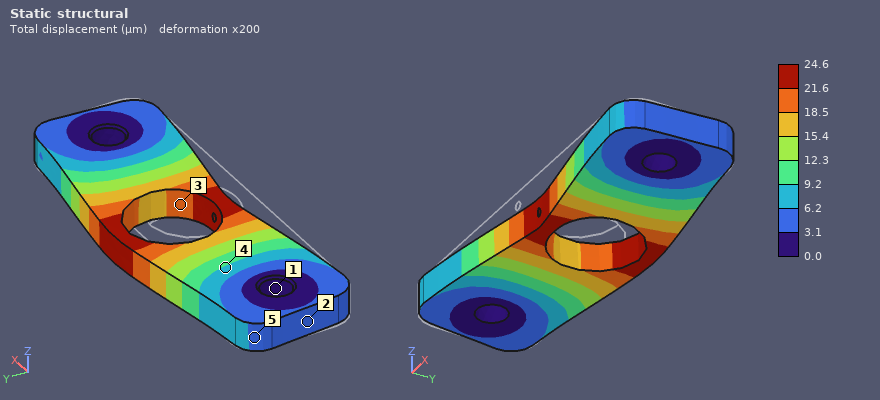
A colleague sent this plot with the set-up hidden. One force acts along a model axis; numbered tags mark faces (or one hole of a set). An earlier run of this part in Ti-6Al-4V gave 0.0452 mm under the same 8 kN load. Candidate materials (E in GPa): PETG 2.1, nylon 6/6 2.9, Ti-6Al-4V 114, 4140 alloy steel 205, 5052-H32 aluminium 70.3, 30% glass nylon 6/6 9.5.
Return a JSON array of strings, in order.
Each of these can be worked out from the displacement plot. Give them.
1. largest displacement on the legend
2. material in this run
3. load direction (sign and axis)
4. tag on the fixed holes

["24.6 µm", "4140 alloy steel", "+Y", "1"]
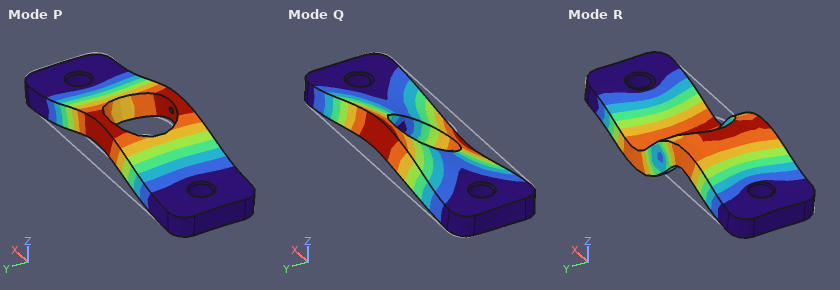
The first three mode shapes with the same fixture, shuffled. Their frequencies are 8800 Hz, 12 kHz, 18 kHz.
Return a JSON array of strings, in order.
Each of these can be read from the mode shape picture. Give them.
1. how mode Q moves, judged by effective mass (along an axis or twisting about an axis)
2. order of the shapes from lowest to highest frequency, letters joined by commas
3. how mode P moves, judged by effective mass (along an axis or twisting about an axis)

["twisting about X", "P, Q, R", "along Z"]
